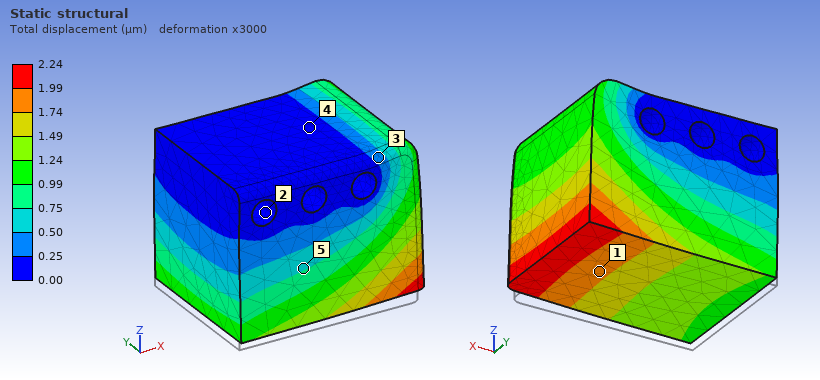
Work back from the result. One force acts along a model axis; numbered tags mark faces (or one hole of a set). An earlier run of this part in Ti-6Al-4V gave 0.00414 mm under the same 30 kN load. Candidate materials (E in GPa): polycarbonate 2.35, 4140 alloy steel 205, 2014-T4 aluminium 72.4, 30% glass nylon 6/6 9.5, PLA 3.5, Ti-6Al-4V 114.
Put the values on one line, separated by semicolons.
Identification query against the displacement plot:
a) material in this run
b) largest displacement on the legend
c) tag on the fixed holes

4140 alloy steel; 2.24 µm; 2
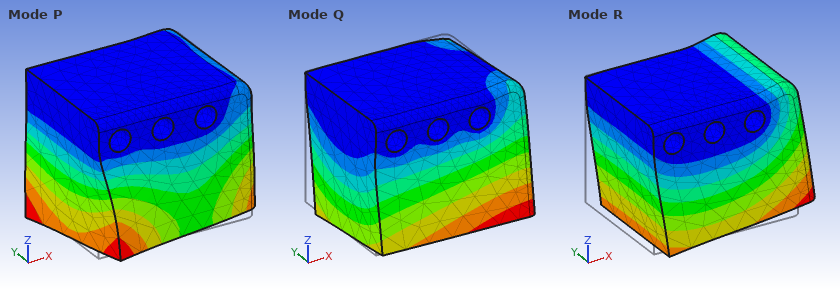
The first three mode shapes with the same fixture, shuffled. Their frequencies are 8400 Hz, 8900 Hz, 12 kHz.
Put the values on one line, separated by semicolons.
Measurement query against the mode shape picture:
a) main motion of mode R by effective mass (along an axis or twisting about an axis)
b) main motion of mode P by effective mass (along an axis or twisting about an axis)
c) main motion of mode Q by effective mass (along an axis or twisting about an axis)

along X; twisting about Z; along Y
